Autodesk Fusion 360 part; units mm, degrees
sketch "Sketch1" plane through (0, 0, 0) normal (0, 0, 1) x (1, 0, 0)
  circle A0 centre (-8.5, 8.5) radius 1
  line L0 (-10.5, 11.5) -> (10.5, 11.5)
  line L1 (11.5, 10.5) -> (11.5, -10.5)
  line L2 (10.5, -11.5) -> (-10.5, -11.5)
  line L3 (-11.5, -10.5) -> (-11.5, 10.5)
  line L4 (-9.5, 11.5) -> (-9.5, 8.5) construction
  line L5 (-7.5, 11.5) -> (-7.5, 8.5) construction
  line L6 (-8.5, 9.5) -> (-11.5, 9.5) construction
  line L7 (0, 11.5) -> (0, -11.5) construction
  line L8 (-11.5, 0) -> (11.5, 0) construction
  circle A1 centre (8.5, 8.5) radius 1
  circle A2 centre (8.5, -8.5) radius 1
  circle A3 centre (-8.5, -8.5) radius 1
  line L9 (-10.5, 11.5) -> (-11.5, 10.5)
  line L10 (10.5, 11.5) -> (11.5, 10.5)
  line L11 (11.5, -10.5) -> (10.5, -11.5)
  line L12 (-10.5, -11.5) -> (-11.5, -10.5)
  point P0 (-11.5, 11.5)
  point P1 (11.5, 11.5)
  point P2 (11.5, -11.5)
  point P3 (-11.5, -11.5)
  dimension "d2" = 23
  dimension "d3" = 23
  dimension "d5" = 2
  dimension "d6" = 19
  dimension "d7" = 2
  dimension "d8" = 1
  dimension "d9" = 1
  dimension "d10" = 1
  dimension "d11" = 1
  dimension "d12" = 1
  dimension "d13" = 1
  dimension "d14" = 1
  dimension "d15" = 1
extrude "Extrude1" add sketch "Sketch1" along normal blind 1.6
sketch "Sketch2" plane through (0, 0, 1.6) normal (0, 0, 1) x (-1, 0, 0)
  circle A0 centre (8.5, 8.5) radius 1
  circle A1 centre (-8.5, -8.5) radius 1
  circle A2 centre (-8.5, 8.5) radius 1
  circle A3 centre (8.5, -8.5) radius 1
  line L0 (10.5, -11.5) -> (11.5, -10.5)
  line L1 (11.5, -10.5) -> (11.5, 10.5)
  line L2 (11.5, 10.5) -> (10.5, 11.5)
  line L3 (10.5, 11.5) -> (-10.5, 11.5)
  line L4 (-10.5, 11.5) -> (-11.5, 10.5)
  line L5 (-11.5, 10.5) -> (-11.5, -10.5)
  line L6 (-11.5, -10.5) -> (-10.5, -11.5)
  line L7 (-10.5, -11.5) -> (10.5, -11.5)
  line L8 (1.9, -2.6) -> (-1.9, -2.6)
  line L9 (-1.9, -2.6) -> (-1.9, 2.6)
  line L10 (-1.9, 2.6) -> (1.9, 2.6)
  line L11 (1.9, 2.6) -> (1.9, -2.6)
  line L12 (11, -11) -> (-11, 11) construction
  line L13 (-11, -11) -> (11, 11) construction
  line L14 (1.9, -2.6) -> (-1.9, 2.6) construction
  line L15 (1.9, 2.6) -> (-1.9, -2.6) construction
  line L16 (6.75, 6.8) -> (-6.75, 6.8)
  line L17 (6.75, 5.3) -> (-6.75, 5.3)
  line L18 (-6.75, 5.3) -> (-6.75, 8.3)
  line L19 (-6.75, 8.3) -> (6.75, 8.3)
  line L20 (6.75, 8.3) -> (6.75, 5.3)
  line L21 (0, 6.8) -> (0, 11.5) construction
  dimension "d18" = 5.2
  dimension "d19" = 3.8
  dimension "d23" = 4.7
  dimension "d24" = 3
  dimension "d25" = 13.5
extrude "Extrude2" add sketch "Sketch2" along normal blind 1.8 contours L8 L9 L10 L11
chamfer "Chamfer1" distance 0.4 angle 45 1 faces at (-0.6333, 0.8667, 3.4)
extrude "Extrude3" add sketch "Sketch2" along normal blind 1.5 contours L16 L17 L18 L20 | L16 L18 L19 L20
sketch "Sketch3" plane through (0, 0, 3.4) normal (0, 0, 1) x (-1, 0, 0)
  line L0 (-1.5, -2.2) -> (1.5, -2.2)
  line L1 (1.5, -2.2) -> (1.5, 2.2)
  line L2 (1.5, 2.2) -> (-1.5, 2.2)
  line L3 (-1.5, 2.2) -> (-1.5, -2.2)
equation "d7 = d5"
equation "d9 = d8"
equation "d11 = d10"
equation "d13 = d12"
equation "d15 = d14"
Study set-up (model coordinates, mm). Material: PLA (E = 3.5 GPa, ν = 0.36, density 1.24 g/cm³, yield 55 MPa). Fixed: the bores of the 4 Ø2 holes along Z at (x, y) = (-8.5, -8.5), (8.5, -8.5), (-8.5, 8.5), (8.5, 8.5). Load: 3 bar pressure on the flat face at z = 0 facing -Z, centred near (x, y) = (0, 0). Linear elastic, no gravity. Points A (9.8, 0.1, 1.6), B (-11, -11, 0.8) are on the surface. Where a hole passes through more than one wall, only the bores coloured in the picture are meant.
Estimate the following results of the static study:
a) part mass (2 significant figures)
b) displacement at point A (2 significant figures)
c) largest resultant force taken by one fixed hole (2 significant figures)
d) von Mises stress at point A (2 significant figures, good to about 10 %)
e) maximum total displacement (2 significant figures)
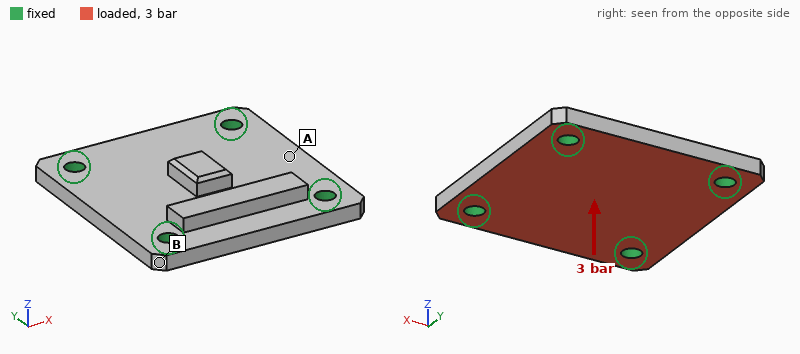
1.1 g
54 µm
40 N
8.4 MPa
90 µm
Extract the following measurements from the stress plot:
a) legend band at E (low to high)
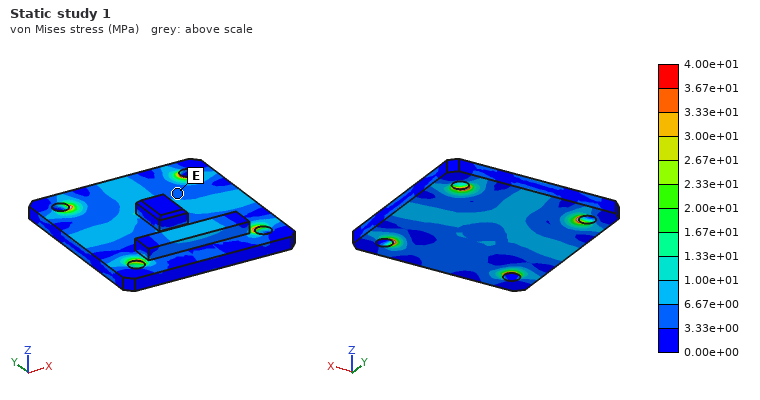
3.33e+00 to 6.67e+00 MPa
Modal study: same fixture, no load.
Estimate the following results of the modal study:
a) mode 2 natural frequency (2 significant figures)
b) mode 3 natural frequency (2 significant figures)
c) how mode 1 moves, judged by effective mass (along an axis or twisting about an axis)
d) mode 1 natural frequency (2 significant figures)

11 kHz
11 kHz
along Z
7100 Hz
